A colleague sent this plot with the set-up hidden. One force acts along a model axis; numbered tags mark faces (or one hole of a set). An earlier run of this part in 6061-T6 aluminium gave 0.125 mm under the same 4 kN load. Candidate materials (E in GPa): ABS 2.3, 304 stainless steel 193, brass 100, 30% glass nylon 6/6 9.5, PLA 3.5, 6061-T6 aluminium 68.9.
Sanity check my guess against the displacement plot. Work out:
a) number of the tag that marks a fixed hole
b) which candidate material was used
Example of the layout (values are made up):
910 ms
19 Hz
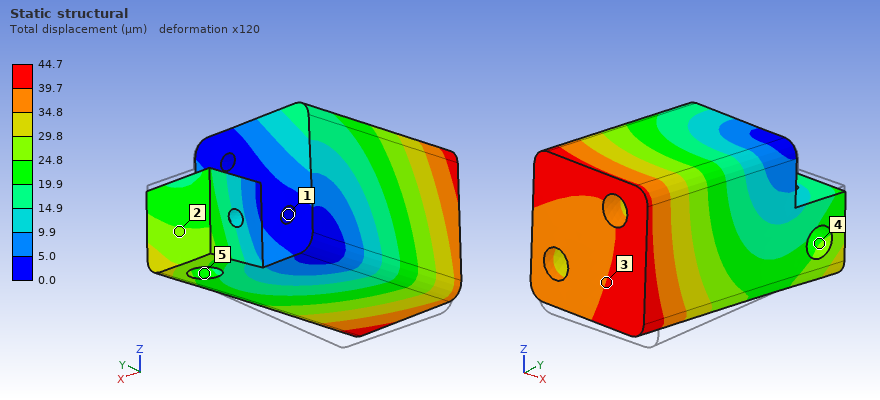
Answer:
1
304 stainless steel
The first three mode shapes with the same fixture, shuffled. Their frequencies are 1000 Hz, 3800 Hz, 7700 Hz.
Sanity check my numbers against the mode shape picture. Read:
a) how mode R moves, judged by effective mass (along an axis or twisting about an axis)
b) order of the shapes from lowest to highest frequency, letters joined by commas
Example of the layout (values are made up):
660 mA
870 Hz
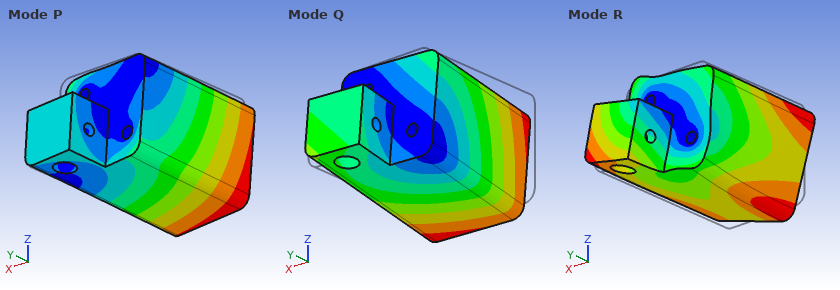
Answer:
twisting about Y
Q, P, R
